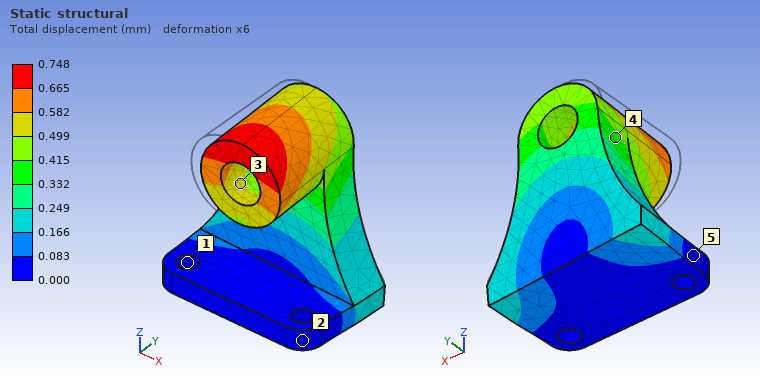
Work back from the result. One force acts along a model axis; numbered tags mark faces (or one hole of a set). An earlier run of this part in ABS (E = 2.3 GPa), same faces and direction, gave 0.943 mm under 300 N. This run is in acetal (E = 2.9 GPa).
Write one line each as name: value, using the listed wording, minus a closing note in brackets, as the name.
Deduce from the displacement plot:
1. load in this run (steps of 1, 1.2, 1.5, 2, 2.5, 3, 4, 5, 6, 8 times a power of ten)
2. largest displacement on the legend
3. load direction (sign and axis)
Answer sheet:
load in this run: 300 N
largest displacement on the legend: 0.748 mm
load direction: +X
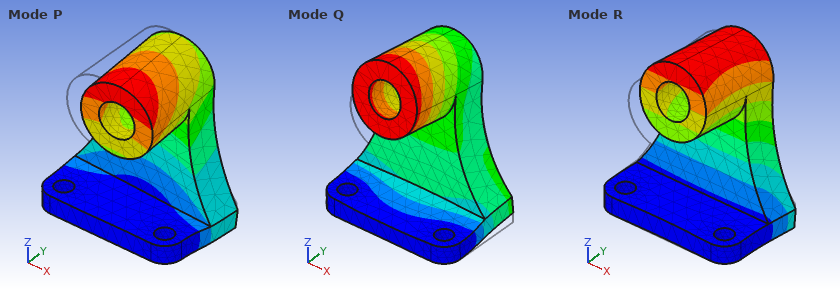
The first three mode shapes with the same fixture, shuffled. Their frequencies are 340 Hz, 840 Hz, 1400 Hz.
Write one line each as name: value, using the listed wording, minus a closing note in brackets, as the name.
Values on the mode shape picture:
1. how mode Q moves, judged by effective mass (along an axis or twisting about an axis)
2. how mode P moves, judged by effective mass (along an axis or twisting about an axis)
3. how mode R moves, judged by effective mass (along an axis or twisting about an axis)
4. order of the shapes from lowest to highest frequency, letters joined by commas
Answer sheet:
how mode Q moves, judged by effective mass: along Z
how mode P moves, judged by effective mass: along X
how mode R moves, judged by effective mass: along Y
order of the shapes from lowest to highest frequency, letters joined by commas: R, P, Q
